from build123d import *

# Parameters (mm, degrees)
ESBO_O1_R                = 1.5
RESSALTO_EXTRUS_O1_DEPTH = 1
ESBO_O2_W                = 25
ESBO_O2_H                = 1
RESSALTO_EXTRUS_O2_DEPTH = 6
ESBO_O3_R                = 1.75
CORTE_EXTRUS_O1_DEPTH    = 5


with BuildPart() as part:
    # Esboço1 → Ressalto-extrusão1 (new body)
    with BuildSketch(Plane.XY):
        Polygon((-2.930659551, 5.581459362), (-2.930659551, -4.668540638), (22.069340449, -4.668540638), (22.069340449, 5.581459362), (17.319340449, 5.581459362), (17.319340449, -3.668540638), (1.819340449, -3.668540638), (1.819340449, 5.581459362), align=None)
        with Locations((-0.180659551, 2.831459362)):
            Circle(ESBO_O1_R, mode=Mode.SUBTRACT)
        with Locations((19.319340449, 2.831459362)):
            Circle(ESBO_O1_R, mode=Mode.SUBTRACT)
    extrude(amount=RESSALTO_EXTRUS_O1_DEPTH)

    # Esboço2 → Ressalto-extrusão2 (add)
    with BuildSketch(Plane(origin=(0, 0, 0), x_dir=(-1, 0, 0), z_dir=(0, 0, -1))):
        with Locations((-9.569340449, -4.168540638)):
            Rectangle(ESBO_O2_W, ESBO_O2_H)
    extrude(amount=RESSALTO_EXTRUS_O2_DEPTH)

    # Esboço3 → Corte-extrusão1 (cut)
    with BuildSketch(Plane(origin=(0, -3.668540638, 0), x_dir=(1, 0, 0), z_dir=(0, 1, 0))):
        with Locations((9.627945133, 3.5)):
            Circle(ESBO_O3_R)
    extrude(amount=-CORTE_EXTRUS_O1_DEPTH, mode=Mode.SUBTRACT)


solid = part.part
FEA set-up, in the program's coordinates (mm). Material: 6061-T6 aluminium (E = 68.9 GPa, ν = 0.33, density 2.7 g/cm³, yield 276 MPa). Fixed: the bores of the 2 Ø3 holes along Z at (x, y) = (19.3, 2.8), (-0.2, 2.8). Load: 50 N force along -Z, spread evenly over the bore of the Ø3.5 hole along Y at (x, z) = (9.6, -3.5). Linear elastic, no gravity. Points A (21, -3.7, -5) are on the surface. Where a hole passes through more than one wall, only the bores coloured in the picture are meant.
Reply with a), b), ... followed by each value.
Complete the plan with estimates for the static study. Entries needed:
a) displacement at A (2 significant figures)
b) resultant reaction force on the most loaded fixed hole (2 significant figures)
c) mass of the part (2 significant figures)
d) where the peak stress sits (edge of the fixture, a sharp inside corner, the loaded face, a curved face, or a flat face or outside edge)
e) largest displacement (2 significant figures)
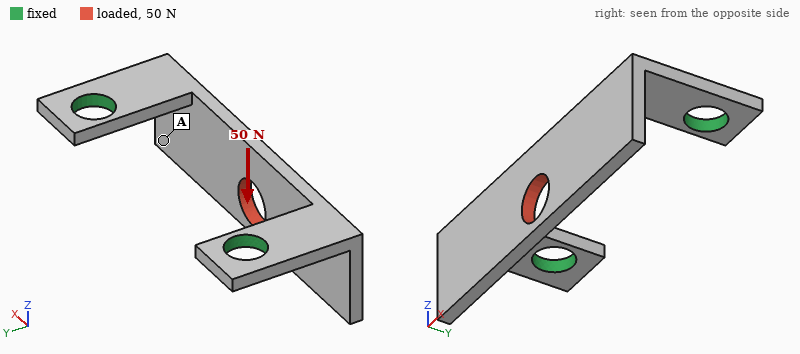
a) 0.095 mm
b) 26 N
c) 0.65 g
d) a flat face or outside edge
e) 0.12 mm
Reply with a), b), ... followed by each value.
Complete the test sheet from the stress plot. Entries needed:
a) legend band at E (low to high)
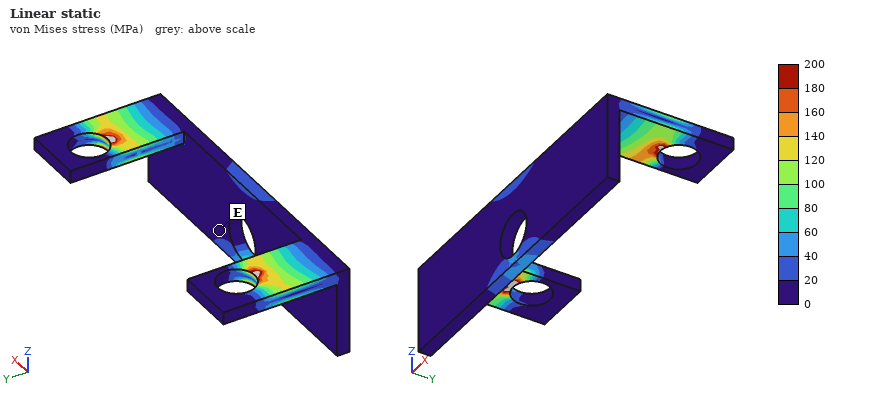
a) 0 to 20 MPa
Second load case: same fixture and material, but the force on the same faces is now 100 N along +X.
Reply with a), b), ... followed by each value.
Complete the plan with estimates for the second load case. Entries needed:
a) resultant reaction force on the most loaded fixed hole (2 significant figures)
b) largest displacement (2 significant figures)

a) 53 N
b) 54 µm
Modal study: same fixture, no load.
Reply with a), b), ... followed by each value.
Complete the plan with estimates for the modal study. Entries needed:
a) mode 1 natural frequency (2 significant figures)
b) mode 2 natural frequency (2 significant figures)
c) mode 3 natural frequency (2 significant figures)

a) 4700 Hz
b) 8800 Hz
c) 12 kHz
